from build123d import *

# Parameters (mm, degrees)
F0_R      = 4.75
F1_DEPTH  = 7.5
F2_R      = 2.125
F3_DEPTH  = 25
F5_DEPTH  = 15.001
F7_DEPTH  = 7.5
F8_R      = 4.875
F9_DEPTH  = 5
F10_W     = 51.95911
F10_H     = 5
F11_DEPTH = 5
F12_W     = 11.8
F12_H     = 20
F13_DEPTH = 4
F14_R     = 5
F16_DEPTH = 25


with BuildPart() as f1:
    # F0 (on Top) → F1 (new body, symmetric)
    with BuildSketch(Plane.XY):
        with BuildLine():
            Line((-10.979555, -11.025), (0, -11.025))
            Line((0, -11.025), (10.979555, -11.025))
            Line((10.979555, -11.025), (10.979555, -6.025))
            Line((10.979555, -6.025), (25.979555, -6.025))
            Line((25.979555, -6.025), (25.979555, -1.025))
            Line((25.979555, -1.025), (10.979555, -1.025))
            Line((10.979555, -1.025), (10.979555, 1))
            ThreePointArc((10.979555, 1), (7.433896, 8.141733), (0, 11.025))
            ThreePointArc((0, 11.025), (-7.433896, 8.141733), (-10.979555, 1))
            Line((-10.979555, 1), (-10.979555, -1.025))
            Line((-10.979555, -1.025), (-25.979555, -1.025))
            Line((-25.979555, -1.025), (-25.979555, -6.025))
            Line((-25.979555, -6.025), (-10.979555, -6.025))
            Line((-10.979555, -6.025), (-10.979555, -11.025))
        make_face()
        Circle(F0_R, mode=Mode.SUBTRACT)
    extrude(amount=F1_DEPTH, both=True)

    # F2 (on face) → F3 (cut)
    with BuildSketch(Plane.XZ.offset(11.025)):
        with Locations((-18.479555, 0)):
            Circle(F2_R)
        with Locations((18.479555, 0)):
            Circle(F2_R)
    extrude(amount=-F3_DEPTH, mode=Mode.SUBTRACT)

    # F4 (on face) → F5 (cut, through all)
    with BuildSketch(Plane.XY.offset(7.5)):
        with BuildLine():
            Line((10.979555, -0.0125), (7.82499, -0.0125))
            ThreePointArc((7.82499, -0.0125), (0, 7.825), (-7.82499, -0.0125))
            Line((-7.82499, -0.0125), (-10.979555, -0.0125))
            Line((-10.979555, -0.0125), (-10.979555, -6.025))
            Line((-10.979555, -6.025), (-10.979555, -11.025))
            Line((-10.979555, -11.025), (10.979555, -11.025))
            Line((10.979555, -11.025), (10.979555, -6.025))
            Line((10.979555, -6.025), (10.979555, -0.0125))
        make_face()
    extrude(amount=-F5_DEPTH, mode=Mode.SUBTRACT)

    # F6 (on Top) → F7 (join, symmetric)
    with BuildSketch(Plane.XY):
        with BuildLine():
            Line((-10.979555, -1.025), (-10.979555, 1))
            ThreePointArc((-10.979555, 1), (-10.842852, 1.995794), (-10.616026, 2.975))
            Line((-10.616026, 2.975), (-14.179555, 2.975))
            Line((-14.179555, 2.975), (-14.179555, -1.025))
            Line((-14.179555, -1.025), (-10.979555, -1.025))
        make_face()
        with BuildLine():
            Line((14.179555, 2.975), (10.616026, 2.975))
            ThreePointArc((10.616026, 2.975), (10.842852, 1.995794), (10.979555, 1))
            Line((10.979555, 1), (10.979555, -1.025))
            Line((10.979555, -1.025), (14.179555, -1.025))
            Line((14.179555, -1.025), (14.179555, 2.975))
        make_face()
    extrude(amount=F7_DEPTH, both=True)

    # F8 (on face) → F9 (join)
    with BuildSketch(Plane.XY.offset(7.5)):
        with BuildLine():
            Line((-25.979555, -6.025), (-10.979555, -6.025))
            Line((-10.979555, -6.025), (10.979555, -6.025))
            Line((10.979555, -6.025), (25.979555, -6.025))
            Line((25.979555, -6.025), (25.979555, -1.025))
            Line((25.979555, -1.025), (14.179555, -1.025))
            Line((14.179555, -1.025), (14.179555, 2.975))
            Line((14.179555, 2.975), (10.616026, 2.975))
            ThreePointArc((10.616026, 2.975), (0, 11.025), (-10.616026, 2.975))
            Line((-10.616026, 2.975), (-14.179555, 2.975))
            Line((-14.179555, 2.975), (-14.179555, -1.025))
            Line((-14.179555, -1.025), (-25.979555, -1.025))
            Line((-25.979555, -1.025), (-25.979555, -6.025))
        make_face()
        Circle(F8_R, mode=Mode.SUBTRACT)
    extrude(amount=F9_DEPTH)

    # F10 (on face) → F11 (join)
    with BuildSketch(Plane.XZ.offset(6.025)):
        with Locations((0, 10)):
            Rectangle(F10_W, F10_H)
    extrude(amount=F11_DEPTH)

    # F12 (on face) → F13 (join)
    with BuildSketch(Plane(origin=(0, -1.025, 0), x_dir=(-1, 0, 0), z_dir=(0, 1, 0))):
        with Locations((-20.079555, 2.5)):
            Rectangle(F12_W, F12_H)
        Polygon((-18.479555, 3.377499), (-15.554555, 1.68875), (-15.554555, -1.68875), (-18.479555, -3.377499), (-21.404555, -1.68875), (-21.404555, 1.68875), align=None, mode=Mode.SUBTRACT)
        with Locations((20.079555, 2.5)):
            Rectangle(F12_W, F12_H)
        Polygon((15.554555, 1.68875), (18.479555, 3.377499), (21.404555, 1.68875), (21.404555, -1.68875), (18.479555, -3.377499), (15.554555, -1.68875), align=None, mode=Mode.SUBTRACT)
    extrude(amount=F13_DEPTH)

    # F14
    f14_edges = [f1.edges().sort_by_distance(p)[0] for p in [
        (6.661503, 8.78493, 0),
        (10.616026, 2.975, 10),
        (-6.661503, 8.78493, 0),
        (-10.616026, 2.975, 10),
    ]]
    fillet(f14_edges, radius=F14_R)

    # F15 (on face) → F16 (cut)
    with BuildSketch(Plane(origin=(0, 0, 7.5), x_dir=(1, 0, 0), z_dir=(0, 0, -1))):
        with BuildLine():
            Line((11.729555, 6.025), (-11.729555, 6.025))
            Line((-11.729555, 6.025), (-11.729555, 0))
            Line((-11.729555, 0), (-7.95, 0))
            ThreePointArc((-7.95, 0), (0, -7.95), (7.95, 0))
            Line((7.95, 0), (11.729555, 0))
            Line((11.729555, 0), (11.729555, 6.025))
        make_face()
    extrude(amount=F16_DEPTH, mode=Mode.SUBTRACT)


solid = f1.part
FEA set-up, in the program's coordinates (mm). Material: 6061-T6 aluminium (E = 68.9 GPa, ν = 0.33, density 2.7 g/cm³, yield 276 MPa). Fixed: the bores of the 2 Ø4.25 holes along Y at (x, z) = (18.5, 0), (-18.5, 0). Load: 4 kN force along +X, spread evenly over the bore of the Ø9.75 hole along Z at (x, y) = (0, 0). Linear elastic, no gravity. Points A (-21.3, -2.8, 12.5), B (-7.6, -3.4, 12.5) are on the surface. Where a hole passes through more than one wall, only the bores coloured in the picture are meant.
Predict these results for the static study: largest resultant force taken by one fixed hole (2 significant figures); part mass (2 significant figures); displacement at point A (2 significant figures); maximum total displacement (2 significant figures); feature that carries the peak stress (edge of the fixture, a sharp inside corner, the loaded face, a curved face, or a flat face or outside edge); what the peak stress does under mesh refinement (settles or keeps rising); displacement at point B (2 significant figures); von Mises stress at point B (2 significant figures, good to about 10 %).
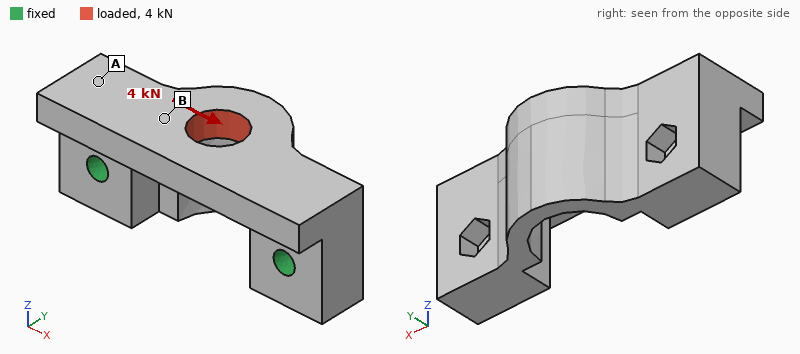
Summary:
2.2 kN
24 g
16 µm
19 µm
edge of the fixture
keeps rising
16 µm
29 MPa
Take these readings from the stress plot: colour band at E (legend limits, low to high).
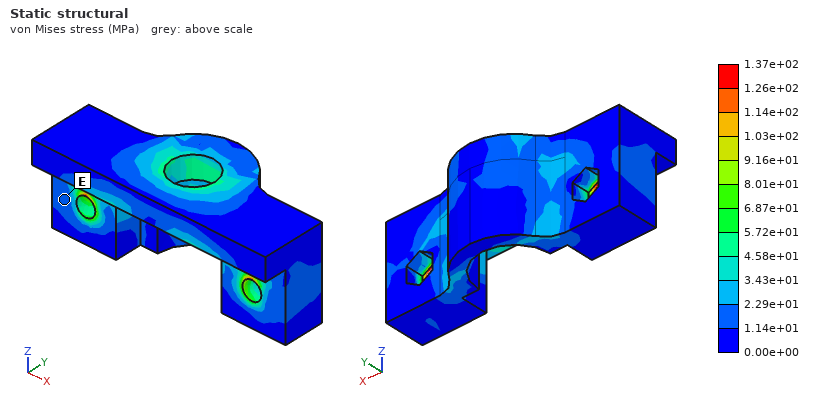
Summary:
1.14e+01 to 2.29e+01 MPa
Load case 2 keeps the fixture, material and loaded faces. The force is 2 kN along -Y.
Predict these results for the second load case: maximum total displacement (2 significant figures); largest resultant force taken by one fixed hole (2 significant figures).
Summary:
45 µm
1.0 kN
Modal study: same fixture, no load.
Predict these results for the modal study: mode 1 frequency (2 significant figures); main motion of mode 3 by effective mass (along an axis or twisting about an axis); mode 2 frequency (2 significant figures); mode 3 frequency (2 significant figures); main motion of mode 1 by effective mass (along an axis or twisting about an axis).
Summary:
11 kHz
along Z
18 kHz
21 kHz
along Y
